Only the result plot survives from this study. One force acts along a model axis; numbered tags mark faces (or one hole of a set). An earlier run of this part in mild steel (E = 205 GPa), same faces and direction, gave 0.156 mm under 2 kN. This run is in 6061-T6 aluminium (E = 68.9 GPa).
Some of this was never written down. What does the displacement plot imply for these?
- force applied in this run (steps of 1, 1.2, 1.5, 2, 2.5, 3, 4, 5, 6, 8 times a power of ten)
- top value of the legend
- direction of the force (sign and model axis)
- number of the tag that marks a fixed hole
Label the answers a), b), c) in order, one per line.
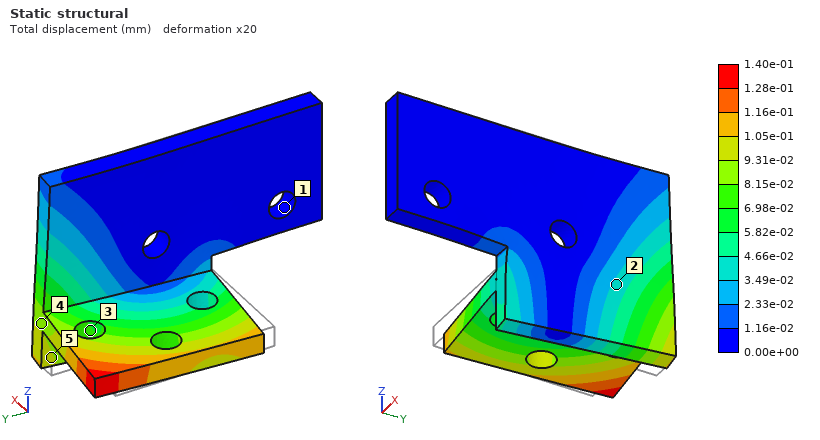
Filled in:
a) 600 N
b) 1.40e-01 mm
c) +Y
d) 1
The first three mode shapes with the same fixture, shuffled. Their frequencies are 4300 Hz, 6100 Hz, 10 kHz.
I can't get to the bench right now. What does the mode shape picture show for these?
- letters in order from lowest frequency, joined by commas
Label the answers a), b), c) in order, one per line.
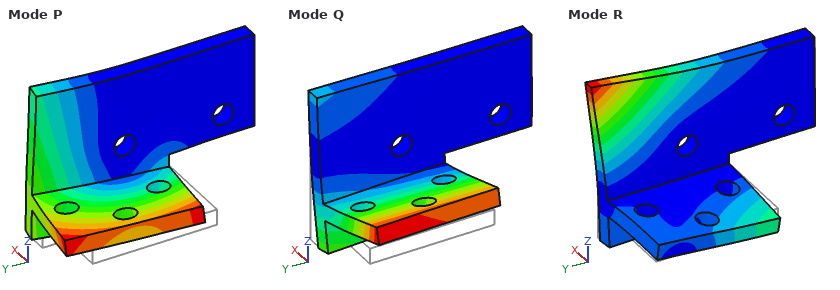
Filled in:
a) Q, P, R
